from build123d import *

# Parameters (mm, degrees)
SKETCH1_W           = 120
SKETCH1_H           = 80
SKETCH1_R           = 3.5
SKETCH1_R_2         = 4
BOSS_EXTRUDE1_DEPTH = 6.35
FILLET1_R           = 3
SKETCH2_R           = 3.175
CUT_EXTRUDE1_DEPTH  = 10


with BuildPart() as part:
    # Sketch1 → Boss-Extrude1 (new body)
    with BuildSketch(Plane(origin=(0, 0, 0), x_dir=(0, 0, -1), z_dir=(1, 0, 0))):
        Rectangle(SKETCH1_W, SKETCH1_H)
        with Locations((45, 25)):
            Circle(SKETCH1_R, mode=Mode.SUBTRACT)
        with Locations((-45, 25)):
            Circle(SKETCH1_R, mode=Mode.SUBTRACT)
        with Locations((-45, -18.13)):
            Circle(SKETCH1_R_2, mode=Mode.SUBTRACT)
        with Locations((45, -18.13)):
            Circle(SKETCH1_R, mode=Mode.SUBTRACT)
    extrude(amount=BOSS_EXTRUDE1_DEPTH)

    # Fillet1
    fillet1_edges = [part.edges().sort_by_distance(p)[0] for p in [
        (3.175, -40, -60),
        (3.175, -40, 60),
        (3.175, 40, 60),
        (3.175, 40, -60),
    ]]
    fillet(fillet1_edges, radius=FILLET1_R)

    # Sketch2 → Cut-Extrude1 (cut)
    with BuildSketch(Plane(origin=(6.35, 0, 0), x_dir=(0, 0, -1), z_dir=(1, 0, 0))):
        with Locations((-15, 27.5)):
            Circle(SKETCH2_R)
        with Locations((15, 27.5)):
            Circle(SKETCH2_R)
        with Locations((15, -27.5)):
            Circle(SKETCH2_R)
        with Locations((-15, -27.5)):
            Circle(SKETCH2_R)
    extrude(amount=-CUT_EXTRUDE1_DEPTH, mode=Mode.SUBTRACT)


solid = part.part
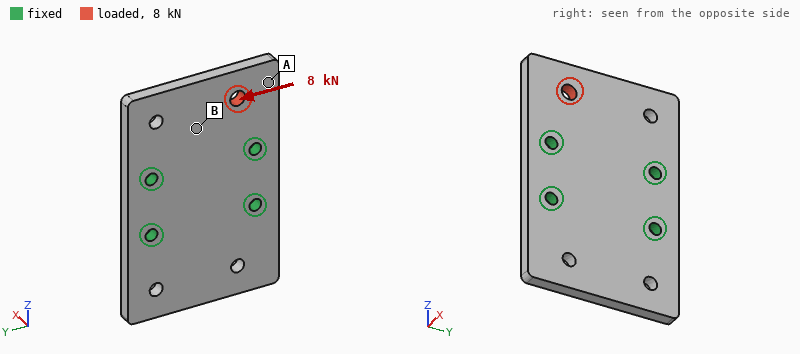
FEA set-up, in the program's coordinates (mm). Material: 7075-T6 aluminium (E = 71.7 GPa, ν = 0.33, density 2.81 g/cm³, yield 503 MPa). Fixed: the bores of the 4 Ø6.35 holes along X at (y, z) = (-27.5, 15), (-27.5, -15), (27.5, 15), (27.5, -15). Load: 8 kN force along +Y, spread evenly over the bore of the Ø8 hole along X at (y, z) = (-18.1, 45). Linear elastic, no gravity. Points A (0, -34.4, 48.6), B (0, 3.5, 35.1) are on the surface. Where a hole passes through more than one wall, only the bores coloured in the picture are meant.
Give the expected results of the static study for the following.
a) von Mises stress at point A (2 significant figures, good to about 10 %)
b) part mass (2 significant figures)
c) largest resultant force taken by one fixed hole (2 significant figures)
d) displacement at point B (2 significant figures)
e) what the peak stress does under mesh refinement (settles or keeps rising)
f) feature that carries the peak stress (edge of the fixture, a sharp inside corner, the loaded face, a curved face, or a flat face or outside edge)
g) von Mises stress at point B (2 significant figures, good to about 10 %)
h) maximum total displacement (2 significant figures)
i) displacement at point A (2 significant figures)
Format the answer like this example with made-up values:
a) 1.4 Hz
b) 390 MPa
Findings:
a) 9.8 MPa
b) 170 g
c) 5.4 kN
d) 17 µm
e) keeps rising
f) edge of the fixture
g) 35 MPa
h) 41 µm
i) 36 µm
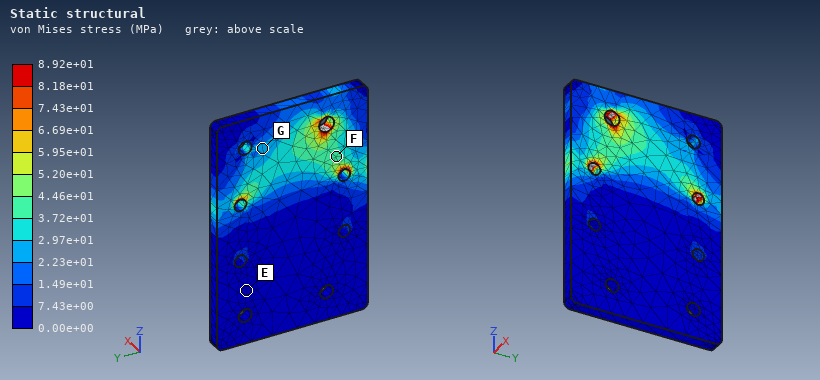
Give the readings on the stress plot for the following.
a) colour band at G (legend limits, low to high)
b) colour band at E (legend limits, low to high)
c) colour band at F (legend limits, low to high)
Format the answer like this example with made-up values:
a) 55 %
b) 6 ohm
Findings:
a) 2.23e+01 to 2.97e+01 MPa
b) 0.00e+00 to 7.43e+00 MPa
c) 3.72e+01 to 4.46e+01 MPa
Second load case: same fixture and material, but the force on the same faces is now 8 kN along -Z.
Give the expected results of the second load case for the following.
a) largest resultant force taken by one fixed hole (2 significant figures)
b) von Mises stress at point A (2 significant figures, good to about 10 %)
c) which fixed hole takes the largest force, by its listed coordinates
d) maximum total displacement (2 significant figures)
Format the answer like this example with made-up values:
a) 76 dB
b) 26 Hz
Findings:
a) 5.3 kN
b) 9.5 MPa
c) (-27.5, 15)
d) 25 µm
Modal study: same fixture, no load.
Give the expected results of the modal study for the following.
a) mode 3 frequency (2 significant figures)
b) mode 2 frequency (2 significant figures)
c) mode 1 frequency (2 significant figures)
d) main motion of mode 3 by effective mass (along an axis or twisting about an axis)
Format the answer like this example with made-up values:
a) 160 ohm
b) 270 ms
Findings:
a) 4100 Hz
b) 2400 Hz
c) 2400 Hz
d) twisting about Z
